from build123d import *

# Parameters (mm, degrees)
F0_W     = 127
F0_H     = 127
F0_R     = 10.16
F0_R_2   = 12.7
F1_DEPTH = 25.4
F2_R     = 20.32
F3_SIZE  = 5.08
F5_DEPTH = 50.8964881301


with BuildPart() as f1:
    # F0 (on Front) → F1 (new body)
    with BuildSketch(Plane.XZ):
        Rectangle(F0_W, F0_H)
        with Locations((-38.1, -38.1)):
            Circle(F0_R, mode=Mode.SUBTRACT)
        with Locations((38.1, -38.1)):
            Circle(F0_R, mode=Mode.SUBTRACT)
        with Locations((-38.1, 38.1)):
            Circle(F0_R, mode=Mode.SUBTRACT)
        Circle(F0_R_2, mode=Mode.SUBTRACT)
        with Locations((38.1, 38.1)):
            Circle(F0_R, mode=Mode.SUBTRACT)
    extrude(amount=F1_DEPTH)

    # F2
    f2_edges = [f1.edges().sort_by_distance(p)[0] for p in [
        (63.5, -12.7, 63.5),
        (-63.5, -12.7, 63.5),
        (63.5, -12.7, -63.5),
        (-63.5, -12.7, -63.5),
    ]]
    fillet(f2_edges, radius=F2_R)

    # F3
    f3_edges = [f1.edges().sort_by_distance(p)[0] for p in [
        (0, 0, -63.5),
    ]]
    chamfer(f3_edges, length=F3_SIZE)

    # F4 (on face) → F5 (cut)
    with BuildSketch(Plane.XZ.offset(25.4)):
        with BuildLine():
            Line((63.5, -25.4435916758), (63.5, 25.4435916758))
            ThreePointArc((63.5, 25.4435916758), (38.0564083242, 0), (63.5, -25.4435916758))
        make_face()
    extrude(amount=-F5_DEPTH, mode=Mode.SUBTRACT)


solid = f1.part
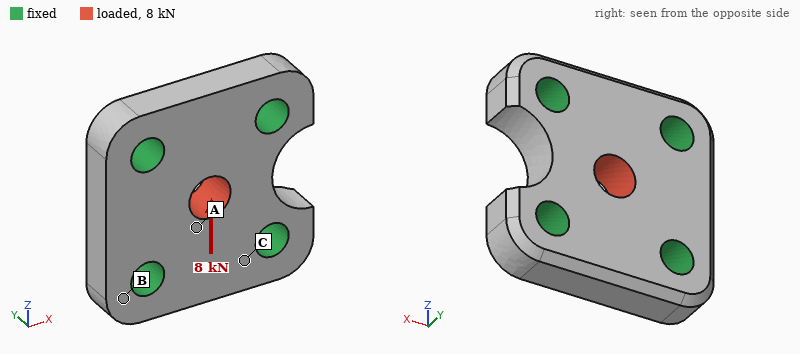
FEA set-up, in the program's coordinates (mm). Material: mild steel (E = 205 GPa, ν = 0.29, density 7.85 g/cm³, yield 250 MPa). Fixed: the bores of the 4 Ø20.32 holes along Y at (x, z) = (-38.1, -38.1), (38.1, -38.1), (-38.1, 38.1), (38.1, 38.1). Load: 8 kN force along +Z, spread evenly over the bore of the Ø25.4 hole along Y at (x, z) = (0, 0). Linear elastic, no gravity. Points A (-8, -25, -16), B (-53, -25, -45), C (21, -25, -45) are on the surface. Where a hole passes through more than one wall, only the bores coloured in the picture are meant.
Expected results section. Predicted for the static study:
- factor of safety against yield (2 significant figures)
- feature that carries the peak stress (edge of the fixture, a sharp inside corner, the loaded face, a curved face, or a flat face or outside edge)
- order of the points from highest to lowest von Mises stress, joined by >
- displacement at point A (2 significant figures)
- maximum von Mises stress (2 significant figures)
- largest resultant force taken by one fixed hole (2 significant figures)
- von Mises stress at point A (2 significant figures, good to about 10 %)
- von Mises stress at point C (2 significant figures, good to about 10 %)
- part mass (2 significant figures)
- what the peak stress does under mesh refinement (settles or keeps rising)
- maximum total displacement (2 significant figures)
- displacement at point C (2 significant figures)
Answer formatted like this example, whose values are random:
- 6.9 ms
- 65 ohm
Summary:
- 36
- the loaded face
- A > C > B
- 0.55 µm
- 6.9 MPa
- 2.2 kN
- 3.5 MPa
- 2.0 MPa
- 2.5 kg
- settles
- 0.70 µm
- 0.17 µm
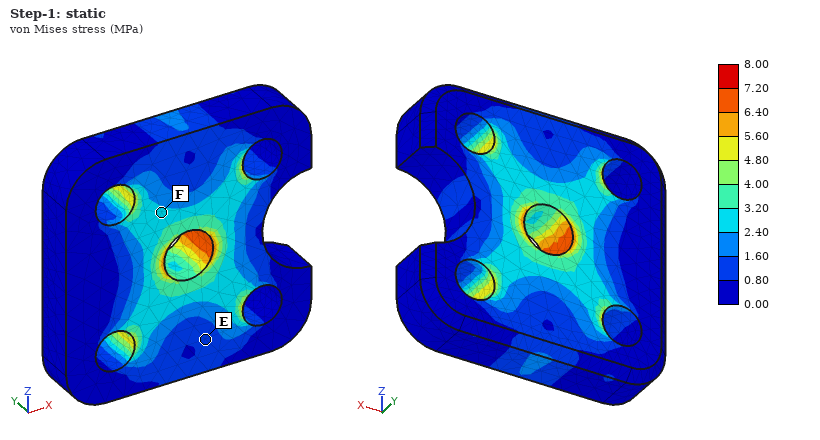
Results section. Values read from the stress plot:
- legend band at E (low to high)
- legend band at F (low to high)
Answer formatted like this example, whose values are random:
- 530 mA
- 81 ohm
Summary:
- 0.80 to 1.60 MPa
- 2.40 to 3.20 MPa
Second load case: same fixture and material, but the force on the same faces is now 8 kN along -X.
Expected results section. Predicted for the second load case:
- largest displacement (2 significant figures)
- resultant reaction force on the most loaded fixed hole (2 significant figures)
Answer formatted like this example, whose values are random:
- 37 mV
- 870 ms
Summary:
- 0.79 µm
- 2.3 kN
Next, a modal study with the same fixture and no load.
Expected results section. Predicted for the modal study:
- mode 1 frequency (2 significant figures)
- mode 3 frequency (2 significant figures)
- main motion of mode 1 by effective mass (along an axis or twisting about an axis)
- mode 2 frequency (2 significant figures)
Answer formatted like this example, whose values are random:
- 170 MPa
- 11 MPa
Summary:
- 15 kHz
- 18 kHz
- along Y
- 18 kHz
